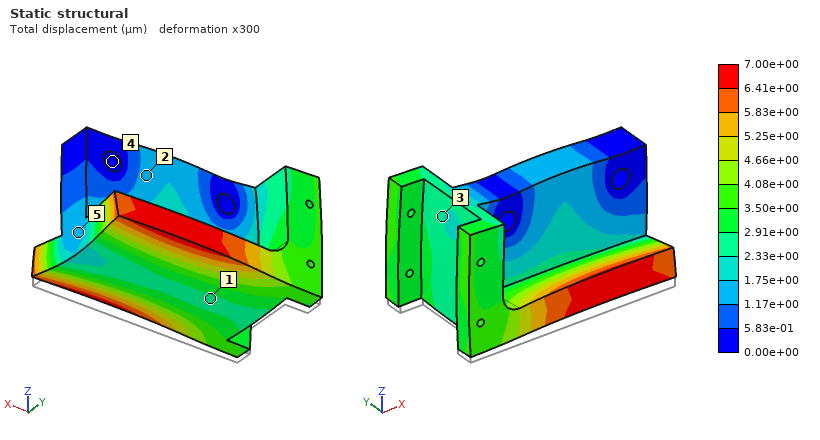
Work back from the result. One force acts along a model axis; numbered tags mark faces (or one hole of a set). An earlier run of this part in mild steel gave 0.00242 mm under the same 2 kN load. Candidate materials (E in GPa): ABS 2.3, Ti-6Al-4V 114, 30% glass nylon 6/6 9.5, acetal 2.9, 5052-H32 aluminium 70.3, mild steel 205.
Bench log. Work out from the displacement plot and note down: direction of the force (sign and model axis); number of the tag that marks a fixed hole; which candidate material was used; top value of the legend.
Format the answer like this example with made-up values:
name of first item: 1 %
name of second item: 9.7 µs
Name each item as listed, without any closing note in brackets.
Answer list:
direction of the force: +Z
number of the tag that marks a fixed hole: 4
which candidate material was used: 5052-H32 aluminium
top value of the legend: 7.00e+00 µm
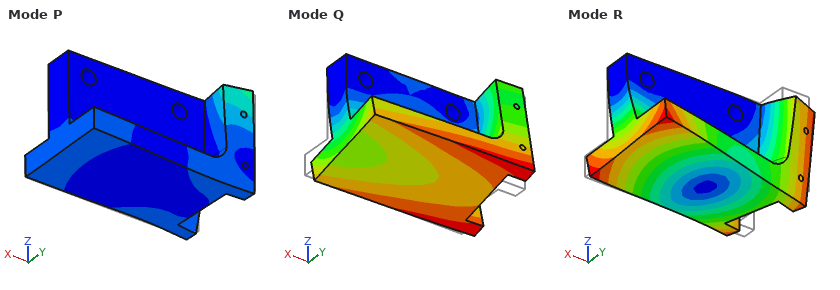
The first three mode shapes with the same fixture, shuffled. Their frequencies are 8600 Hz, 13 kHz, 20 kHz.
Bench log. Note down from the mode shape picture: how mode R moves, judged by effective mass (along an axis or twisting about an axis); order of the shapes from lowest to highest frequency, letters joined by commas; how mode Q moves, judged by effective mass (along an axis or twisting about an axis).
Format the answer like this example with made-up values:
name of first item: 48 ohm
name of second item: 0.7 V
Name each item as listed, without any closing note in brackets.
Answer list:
how mode R moves, judged by effective mass: twisting about Z
order of the shapes from lowest to highest frequency, letters joined by commas: Q, R, P
how mode Q moves, judged by effective mass: along Y
